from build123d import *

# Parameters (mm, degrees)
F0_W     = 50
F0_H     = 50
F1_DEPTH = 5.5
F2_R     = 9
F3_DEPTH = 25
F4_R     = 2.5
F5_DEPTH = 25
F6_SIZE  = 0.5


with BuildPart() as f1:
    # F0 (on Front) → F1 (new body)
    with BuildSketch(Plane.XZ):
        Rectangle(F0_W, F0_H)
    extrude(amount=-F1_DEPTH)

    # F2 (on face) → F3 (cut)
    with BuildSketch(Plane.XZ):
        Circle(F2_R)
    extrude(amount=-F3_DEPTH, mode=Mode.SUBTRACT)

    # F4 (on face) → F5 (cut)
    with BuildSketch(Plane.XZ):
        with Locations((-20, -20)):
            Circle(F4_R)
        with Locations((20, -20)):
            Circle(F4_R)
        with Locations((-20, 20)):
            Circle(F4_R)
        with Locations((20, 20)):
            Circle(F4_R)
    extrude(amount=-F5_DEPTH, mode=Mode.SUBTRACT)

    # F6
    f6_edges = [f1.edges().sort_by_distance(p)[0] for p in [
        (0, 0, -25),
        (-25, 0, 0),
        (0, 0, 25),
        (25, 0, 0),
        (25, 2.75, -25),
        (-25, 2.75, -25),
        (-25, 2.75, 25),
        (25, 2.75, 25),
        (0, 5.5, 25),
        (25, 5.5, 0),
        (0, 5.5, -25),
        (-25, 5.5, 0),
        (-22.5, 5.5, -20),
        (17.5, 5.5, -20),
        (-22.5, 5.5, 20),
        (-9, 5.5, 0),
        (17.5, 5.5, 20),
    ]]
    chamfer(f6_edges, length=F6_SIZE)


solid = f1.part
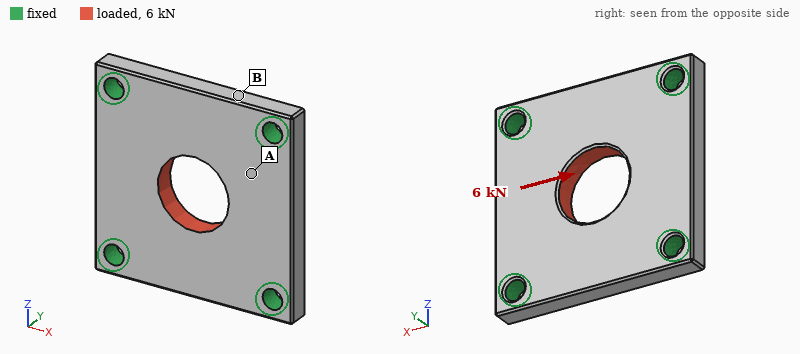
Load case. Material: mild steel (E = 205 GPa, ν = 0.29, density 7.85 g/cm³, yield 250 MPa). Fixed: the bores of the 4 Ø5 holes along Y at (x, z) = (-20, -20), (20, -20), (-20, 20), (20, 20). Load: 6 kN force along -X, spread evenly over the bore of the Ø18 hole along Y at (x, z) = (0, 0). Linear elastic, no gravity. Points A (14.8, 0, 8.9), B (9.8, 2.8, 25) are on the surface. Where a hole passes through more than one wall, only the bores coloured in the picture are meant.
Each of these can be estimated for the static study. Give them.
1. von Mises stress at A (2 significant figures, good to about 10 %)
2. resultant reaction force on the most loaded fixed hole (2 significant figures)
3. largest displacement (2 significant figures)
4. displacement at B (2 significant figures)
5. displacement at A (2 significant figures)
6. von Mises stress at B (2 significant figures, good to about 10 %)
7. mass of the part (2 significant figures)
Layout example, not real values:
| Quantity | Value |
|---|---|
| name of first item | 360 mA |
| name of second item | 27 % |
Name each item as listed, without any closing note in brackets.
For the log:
| Quantity | Value |
|---|---|
| von Mises stress at A | 21 MPa |
| resultant reaction force on the most loaded fixed hole | 1.6 kN |
| largest displacement | 3.4 µm |
| displacement at B | 0.55 µm |
| displacement at A | 2.0 µm |
| von Mises stress at B | 9.2 MPa |
| mass of the part | 93 g |
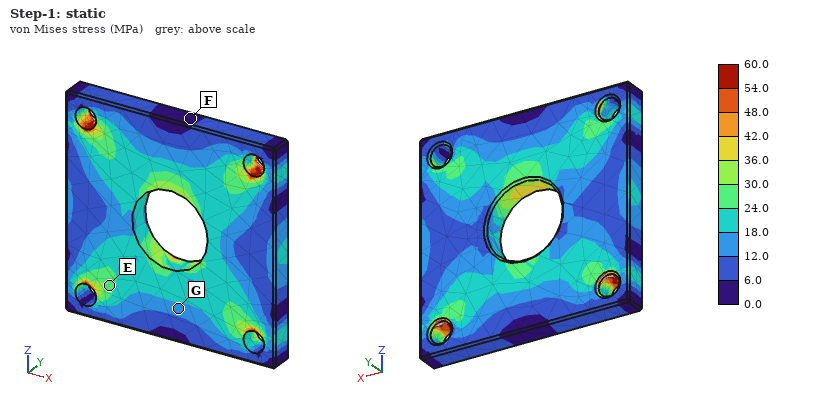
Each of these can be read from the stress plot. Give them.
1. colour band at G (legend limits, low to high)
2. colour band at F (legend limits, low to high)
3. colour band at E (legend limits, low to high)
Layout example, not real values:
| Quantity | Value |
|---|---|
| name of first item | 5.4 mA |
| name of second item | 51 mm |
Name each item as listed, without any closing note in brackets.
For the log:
| Quantity | Value |
|---|---|
| colour band at G | 12.0 to 18.0 MPa |
| colour band at F | 0.0 to 6.0 MPa |
| colour band at E | 24.0 to 30.0 MPa |
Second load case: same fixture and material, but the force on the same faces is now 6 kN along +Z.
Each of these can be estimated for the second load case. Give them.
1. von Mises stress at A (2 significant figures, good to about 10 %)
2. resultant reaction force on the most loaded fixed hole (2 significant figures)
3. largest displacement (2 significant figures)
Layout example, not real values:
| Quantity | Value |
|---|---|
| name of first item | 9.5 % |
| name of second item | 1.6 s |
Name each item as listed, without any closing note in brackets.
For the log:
| Quantity | Value |
|---|---|
| von Mises stress at A | 20 MPa |
| resultant reaction force on the most loaded fixed hole | 1.6 kN |
| largest displacement | 3.4 µm |
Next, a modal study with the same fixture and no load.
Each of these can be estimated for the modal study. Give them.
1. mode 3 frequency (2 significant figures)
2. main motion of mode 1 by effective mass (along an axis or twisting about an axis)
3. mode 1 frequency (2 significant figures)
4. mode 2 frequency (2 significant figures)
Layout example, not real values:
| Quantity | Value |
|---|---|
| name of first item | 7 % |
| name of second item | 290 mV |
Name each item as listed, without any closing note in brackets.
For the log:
| Quantity | Value |
|---|---|
| mode 3 frequency | 18 kHz |
| main motion of mode 1 by effective mass | along Y |
| mode 1 frequency | 13 kHz |
| mode 2 frequency | 18 kHz |
